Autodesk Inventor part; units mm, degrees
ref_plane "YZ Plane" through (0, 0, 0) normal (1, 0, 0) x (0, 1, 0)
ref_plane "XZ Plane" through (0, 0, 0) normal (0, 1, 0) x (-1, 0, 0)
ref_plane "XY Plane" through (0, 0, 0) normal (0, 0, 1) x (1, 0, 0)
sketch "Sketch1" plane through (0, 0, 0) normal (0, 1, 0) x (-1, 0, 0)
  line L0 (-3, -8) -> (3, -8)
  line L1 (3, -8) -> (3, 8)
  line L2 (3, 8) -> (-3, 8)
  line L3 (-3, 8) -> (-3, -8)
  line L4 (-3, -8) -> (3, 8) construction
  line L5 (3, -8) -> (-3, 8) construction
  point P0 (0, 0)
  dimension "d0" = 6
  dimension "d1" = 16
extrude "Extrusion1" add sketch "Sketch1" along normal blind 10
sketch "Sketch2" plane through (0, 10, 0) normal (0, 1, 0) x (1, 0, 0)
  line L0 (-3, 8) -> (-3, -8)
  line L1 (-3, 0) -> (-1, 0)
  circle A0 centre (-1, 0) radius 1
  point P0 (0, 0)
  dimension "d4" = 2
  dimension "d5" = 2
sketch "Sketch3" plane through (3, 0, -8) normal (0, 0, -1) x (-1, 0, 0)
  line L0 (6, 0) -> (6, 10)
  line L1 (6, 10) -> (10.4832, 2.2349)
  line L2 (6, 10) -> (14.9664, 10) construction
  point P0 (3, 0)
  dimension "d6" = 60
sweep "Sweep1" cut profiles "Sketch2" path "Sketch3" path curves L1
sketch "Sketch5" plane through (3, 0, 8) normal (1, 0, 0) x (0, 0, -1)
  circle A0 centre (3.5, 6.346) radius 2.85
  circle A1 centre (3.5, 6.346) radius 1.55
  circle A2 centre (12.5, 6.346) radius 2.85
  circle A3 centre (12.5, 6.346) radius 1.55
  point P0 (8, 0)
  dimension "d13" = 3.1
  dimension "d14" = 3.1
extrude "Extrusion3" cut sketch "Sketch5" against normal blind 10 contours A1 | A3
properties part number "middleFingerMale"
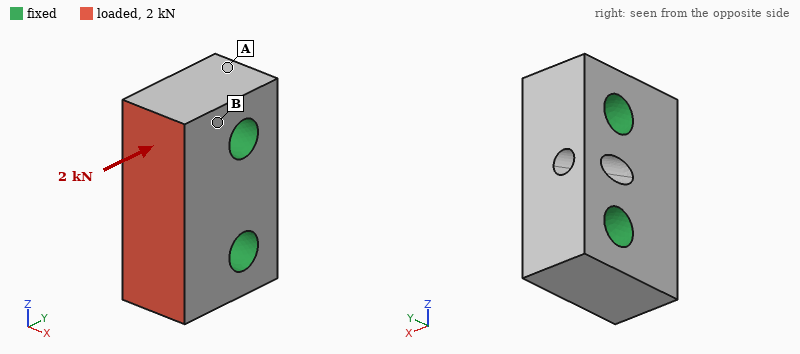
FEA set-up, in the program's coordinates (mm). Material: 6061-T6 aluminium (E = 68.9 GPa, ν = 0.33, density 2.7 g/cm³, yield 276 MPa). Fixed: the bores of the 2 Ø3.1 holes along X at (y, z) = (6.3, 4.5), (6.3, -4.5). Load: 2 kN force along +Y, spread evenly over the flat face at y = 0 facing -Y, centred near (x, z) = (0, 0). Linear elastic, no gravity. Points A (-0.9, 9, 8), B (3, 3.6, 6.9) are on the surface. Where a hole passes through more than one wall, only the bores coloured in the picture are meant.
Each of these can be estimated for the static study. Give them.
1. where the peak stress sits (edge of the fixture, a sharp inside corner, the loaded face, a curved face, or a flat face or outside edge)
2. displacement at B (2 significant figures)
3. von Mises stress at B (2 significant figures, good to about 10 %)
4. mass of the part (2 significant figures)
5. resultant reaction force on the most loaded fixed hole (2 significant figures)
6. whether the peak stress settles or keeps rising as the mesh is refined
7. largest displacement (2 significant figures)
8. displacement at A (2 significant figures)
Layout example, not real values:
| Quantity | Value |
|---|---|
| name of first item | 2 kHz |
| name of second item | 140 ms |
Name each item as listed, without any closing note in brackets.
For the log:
| Quantity | Value |
|---|---|
| where the peak stress sits | edge of the fixture |
| displacement at B | 1.1 µm |
| von Mises stress at B | 17 MPa |
| mass of the part | 2.3 g |
| resultant reaction force on the most loaded fixed hole | 1.0 kN |
| whether the peak stress settles or keeps rising as the mesh is refined | keeps rising |
| largest displacement | 2.3 µm |
| displacement at A | 0.34 µm |
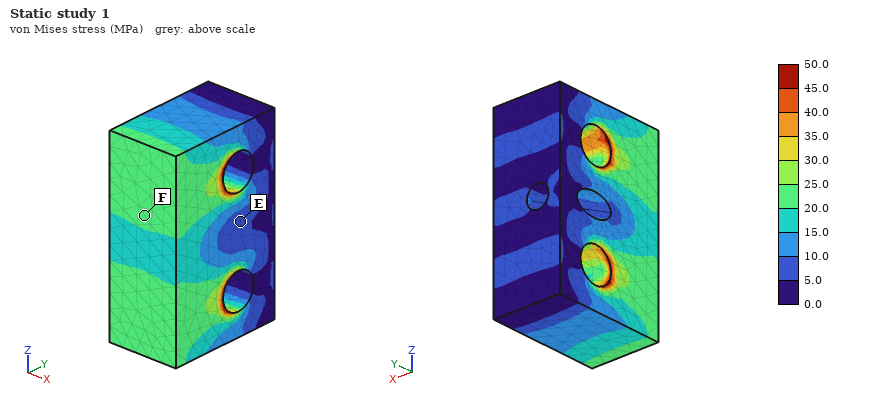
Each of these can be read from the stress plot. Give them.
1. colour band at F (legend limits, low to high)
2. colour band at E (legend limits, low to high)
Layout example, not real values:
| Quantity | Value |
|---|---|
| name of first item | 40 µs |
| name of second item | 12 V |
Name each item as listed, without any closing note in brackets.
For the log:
| Quantity | Value |
|---|---|
| colour band at F | 20.0 to 25.0 MPa |
| colour band at E | 5.0 to 10.0 MPa |
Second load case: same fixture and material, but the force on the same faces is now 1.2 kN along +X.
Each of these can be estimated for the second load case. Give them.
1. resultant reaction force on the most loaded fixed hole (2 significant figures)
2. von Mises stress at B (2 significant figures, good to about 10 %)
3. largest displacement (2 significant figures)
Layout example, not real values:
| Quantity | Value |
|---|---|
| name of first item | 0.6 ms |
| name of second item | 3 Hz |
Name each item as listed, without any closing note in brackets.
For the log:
| Quantity | Value |
|---|---|
| resultant reaction force on the most loaded fixed hole | 600 N |
| von Mises stress at B | 38 MPa |
| largest displacement | 8.7 µm |
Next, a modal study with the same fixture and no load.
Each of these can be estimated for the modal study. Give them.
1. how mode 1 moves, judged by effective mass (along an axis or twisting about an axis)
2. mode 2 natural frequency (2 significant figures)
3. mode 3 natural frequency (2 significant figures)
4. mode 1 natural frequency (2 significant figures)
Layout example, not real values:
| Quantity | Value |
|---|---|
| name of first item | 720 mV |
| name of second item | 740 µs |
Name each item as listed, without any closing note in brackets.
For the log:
| Quantity | Value |
|---|---|
| how mode 1 moves, judged by effective mass | along X |
| mode 2 natural frequency | 110 kHz |
| mode 3 natural frequency | 110 kHz |
| mode 1 natural frequency | 91 kHz |
